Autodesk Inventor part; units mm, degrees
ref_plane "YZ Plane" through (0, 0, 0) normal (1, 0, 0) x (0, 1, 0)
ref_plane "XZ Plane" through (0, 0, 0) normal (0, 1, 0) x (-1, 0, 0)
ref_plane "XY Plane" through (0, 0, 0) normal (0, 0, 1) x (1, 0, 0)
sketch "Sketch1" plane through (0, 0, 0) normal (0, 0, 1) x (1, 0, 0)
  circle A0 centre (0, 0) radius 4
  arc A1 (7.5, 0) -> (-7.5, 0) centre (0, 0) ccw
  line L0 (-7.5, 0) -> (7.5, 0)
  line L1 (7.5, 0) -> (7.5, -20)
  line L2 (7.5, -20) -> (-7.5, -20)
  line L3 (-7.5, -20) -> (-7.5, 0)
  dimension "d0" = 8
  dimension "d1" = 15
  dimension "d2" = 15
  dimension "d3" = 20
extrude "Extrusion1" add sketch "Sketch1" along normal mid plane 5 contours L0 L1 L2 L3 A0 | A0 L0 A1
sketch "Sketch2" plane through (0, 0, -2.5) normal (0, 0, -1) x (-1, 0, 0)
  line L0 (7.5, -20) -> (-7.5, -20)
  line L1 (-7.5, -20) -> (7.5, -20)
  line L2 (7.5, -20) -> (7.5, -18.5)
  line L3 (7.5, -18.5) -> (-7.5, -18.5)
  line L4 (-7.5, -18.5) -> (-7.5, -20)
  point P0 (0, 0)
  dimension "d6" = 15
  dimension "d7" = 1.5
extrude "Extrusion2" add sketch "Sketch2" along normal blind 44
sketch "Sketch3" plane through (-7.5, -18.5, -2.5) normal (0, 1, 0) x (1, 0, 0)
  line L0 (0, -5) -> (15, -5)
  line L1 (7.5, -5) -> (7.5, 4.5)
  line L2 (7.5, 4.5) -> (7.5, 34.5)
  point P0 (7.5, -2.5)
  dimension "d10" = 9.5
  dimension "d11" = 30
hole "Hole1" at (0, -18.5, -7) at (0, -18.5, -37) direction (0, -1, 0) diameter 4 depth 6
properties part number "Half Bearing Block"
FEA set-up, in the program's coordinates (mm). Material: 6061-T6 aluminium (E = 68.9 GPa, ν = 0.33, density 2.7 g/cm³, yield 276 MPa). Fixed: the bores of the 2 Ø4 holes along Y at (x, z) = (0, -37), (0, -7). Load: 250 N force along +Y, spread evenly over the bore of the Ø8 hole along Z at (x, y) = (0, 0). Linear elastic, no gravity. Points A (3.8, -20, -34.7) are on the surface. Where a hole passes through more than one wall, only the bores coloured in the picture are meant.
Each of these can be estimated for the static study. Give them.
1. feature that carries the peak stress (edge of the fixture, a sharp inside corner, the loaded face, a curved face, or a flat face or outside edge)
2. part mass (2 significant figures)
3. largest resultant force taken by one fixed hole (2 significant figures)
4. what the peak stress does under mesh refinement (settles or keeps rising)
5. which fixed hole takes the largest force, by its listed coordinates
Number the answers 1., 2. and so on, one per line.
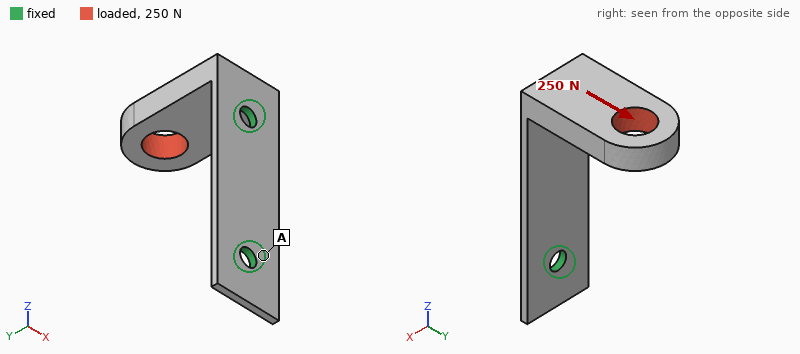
1. edge of the fixture
2. 7.1 g
3. 250 N
4. keeps rising
5. (0, -7)
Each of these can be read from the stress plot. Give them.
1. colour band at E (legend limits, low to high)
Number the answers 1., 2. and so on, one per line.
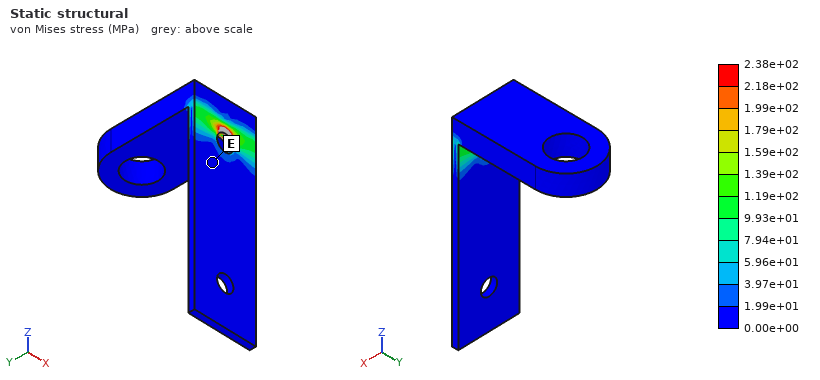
1. 0.00e+00 to 1.99e+01 MPa
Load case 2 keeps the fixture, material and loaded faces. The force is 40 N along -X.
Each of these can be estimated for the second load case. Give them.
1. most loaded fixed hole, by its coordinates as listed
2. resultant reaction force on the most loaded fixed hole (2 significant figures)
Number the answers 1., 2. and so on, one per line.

1. (0, -7)
2. 45 N
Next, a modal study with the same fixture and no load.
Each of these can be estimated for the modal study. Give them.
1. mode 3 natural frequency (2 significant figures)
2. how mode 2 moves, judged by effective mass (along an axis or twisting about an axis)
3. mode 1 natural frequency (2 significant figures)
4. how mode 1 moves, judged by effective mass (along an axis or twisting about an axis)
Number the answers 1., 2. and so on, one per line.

1. 9500 Hz
2. along X
3. 1400 Hz
4. along Z
